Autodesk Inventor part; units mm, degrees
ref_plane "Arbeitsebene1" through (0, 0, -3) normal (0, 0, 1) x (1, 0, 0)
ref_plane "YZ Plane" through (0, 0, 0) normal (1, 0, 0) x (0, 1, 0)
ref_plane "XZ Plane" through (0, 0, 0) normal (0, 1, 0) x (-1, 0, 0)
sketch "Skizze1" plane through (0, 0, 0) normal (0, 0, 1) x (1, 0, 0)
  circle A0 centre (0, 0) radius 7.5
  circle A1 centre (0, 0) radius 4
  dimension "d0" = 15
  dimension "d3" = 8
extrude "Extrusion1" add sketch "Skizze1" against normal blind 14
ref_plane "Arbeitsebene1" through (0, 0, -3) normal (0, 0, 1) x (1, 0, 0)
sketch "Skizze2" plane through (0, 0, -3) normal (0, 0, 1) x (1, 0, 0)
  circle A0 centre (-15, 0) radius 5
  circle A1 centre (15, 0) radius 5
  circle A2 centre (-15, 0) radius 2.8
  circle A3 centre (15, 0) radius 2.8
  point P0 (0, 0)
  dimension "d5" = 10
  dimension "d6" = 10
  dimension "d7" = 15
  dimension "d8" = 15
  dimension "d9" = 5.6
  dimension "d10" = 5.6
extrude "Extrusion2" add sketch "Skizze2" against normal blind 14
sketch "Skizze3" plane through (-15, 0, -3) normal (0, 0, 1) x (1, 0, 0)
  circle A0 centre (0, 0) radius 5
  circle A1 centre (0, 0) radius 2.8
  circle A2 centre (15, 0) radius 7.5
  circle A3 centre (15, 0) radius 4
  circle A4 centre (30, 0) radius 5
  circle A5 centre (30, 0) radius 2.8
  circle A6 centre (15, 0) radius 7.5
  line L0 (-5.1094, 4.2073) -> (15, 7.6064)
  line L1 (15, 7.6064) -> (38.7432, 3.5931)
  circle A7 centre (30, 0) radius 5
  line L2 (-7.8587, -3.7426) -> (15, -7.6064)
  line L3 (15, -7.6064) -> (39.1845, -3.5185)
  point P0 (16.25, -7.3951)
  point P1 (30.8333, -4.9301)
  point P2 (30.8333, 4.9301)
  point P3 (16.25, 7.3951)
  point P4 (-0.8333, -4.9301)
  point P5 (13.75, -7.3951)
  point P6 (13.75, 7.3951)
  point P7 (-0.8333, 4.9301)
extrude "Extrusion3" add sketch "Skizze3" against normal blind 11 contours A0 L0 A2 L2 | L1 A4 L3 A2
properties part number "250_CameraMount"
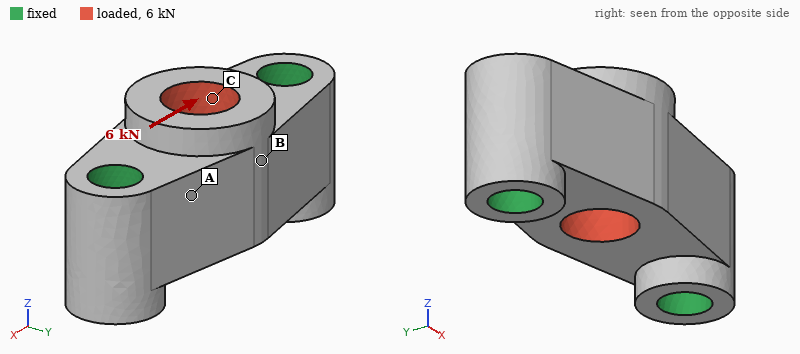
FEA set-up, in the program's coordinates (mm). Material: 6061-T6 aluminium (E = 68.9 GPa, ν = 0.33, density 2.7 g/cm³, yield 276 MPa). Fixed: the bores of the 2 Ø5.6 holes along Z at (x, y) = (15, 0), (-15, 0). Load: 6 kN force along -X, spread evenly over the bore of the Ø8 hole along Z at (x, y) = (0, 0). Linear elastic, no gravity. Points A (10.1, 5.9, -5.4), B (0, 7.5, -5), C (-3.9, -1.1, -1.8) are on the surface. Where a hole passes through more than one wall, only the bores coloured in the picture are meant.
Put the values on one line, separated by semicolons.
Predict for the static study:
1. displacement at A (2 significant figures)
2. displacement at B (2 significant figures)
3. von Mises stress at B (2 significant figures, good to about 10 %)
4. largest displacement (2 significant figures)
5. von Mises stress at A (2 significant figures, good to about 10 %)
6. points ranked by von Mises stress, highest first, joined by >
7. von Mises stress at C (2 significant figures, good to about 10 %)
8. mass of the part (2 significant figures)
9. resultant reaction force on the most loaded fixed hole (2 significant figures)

2.2 µm; 3.3 µm; 8.1 MPa; 6.3 µm; 17 MPa; C > A > B; 27 MPa; 13 g; 3.0 kN
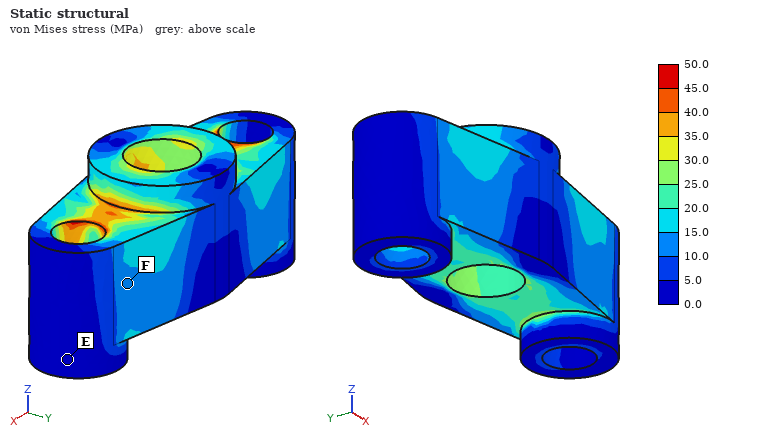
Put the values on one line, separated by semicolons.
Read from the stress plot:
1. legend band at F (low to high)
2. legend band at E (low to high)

10.0 to 15.0 MPa; 0.0 to 5.0 MPa
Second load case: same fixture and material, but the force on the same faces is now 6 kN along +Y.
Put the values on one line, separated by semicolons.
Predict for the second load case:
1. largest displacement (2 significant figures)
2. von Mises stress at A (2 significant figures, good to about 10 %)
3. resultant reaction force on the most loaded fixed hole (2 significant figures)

23 µm; 24 MPa; 3.0 kN
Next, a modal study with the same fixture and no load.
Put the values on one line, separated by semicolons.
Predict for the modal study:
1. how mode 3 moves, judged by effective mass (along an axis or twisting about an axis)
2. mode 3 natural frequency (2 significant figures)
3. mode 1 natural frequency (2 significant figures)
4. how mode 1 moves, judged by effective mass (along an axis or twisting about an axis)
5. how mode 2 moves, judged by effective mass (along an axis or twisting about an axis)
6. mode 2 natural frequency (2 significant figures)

along Y; 49 kHz; 39 kHz; along Y; along Z; 45 kHz
